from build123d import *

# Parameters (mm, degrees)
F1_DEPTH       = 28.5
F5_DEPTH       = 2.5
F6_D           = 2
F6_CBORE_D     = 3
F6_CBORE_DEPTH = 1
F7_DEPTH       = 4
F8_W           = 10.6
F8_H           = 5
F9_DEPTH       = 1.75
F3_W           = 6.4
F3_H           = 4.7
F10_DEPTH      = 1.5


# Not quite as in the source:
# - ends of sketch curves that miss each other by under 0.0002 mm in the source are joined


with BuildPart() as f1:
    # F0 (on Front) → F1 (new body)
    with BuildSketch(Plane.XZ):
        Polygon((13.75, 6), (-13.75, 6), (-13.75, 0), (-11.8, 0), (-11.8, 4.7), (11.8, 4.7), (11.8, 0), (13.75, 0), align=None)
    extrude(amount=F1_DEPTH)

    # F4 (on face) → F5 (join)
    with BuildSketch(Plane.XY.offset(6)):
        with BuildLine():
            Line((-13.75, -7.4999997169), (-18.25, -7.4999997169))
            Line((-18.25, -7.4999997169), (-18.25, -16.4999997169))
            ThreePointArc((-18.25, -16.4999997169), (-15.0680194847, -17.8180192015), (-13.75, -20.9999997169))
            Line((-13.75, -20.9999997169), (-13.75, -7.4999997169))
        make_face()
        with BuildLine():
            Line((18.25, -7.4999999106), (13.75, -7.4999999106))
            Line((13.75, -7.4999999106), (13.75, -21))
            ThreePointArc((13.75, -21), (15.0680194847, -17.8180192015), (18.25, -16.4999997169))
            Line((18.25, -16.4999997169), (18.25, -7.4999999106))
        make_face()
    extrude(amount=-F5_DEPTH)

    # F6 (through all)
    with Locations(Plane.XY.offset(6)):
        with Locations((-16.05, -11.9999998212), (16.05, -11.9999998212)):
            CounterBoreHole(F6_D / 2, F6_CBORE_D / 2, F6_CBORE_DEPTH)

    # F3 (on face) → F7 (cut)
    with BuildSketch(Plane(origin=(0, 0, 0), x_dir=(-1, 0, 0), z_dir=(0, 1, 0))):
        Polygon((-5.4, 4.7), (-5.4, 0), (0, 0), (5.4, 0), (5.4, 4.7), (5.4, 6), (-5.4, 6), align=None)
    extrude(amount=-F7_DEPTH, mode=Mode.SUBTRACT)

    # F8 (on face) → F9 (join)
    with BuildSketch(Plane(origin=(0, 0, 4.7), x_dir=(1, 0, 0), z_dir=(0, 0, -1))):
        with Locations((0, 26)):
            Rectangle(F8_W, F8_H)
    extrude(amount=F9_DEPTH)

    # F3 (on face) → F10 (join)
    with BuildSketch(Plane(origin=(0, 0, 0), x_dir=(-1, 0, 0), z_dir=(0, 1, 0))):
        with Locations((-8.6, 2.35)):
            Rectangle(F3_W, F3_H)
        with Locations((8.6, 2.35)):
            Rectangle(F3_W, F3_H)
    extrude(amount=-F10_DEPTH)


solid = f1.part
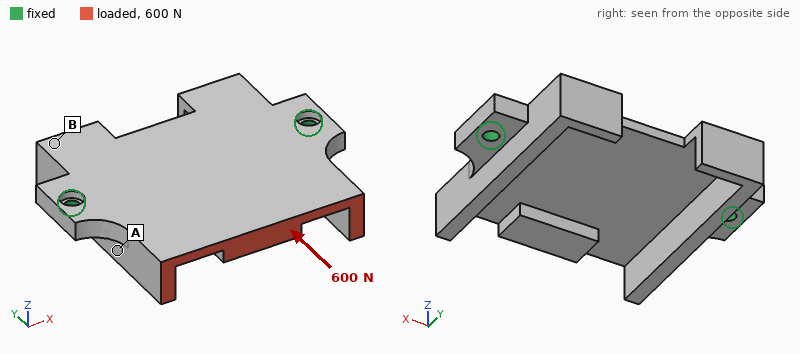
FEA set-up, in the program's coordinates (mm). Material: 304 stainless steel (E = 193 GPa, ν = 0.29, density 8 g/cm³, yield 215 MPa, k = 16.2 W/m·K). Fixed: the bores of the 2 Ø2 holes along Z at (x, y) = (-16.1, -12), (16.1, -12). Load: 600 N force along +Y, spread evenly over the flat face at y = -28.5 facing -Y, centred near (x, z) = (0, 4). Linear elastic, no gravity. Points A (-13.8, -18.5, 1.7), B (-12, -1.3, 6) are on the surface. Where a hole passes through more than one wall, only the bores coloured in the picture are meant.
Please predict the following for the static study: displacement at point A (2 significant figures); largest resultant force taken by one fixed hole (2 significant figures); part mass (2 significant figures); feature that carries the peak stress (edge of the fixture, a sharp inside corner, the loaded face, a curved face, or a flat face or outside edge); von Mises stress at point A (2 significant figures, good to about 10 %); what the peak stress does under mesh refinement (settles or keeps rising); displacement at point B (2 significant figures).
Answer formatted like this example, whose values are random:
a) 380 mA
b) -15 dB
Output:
a) 1.5 µm
b) 310 N
c) 15 g
d) edge of the fixture
e) 16 MPa
f) keeps rising
g) 1.5 µm
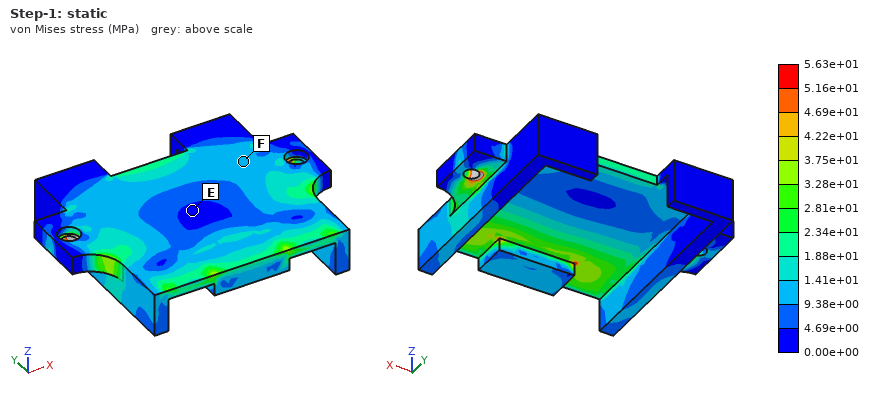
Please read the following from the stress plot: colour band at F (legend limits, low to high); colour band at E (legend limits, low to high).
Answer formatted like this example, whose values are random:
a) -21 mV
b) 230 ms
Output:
a) 9.38e+00 to 1.41e+01 MPa
b) 0.00e+00 to 4.69e+00 MPa
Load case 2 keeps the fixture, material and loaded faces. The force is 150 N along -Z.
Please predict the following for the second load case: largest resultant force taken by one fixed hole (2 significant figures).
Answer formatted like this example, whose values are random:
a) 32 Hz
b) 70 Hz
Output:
a) 110 N
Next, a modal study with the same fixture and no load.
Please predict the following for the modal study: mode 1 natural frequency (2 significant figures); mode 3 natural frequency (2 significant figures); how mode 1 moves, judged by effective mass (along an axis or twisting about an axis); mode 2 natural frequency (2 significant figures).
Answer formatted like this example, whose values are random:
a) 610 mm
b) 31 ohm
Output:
a) 4300 Hz
b) 7400 Hz
c) along Z
d) 7100 Hz
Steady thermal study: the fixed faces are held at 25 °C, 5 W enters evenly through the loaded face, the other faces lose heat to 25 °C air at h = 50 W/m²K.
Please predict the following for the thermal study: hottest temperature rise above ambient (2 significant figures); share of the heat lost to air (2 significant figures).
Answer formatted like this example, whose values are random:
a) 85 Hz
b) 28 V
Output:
a) 77 K
b) 61 %
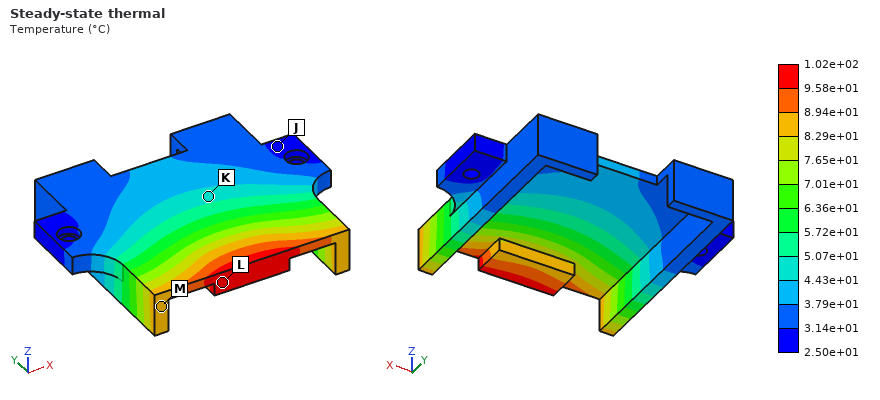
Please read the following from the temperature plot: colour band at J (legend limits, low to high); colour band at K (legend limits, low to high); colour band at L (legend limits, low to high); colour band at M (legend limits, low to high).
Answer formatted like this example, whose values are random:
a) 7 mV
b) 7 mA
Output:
a) 2.50e+01 to 3.14e+01 °C
b) 4.43e+01 to 5.07e+01 °C
c) 9.58e+01 to 1.02e+02 °C
d) 8.29e+01 to 8.94e+01 °C
